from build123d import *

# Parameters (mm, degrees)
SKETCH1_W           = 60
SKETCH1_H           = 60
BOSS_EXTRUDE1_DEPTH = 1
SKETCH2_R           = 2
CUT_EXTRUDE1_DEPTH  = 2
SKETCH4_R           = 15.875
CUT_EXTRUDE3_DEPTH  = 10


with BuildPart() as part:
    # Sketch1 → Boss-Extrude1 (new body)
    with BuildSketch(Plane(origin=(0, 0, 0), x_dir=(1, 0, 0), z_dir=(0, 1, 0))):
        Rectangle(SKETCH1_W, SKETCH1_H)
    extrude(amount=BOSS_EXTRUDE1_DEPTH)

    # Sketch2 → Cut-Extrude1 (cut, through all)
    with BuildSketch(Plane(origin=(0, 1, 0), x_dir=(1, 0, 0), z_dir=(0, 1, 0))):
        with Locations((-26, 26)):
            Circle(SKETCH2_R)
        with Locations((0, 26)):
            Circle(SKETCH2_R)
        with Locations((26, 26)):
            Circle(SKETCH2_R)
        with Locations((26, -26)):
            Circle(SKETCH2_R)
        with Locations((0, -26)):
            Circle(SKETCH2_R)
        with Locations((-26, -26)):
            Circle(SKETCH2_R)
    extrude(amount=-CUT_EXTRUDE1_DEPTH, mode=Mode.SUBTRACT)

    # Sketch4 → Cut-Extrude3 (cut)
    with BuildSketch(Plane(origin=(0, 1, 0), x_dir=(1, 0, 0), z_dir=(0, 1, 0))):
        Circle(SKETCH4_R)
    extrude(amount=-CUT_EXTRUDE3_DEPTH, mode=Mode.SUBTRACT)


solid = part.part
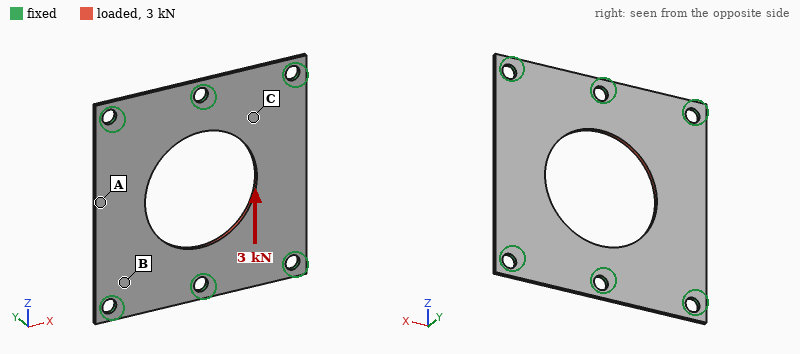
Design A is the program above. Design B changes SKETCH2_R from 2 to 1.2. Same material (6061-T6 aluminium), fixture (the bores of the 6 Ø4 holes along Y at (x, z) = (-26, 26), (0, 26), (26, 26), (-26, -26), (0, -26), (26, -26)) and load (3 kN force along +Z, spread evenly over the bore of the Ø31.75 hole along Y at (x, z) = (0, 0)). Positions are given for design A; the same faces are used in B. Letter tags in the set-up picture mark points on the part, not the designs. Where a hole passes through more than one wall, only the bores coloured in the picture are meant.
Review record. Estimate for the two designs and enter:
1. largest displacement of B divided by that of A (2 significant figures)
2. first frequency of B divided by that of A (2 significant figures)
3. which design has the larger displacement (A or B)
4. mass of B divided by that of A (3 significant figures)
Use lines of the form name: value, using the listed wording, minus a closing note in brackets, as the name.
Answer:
largest displacement of B divided by that of A: 1.1
first frequency of B divided by that of A: 0.91
which design has the larger displacement: B
mass of B divided by that of A: 1.02
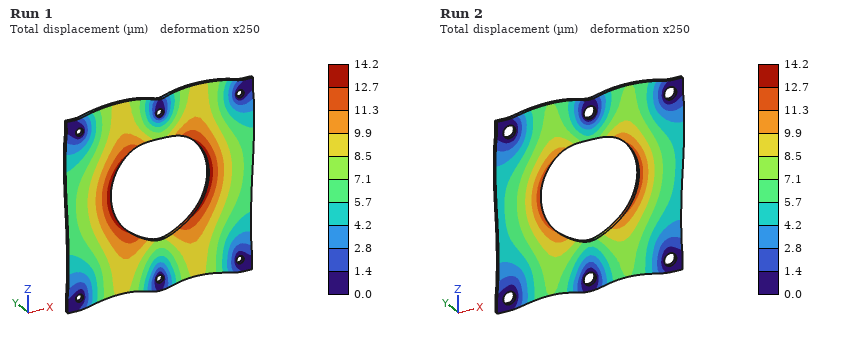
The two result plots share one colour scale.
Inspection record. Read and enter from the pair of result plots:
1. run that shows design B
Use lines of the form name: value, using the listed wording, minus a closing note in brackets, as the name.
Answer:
run that shows design B: Run 1
